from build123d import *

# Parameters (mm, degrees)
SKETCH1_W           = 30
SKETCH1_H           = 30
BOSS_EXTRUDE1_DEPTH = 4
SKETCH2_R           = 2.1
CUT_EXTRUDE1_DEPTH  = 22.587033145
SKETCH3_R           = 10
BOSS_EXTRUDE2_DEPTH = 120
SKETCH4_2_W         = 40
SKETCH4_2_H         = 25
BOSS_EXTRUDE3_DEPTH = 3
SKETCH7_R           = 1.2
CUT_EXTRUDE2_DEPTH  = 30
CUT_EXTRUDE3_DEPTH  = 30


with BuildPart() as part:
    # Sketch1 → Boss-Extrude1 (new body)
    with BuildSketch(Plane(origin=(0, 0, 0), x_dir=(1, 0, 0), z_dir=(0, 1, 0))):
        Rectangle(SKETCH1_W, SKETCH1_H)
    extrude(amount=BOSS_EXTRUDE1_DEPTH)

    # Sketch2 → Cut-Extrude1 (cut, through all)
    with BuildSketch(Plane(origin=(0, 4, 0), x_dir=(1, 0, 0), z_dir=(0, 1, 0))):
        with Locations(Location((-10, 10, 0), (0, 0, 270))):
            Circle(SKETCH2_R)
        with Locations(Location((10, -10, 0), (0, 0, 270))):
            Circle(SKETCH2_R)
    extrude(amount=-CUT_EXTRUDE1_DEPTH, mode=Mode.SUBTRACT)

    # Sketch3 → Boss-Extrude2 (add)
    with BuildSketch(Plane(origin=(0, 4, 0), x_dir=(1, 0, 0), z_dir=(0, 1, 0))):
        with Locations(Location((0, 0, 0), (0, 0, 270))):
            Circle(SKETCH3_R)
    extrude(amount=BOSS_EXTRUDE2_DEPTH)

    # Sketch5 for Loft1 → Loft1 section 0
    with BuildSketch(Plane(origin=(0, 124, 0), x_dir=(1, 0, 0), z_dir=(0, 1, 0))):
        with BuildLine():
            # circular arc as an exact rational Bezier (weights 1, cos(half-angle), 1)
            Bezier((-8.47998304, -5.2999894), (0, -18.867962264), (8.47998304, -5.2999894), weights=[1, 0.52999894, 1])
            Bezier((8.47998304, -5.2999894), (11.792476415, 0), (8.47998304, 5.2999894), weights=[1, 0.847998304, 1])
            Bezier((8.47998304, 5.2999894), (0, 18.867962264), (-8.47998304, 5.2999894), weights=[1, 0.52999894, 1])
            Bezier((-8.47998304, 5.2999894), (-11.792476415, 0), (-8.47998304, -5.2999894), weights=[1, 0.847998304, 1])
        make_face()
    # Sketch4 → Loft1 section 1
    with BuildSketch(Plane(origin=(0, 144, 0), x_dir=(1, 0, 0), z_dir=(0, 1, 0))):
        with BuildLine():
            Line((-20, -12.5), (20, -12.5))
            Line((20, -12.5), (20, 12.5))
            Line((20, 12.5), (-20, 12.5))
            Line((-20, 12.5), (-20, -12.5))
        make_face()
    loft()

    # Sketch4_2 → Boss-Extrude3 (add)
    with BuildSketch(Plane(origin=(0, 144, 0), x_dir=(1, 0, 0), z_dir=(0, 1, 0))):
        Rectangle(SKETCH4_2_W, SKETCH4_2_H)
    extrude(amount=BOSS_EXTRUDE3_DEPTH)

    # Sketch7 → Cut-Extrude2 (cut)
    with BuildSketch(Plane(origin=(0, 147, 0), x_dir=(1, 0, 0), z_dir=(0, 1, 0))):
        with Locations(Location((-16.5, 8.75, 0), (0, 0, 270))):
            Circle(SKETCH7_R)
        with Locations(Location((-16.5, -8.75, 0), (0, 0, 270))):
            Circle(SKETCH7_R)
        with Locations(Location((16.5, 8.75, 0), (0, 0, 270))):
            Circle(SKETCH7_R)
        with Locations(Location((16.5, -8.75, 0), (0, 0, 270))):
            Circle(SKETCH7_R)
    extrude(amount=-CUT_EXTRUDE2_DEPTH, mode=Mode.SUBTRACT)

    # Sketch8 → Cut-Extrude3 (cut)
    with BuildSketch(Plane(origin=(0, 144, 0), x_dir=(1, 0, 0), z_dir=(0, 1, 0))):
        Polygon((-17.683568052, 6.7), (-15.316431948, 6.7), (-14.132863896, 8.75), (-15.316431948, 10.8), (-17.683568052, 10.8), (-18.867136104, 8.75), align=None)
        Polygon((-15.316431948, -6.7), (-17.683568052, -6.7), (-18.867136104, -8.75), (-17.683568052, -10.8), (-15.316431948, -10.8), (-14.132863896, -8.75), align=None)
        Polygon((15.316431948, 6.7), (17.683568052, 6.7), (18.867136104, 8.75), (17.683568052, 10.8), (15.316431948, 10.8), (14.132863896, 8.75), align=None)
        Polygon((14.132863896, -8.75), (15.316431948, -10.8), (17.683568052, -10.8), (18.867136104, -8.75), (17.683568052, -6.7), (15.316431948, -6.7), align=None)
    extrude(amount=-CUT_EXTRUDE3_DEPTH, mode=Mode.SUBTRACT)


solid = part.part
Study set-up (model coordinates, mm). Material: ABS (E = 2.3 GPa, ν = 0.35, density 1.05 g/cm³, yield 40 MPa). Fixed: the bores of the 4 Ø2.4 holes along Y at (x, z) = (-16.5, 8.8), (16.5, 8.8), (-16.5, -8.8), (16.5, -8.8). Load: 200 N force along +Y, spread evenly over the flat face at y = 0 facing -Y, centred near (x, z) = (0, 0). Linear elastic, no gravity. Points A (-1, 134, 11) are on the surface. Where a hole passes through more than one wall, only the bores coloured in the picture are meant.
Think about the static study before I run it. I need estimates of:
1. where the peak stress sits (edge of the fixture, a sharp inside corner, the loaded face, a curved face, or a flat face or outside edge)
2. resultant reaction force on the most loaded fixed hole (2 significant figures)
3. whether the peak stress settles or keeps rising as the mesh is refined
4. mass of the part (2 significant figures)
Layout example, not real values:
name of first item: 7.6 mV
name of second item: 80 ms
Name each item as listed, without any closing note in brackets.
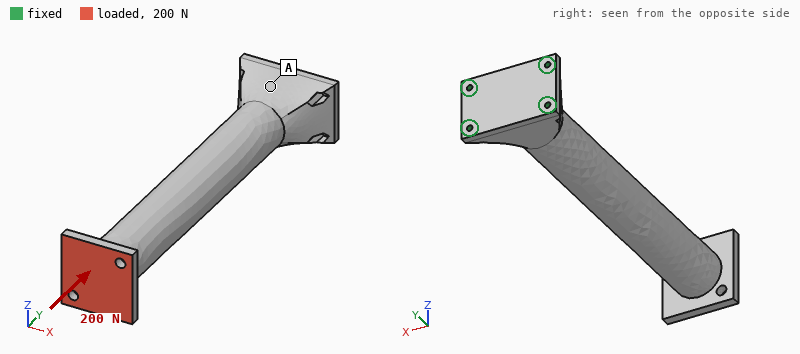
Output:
where the peak stress sits: edge of the fixture
resultant reaction force on the most loaded fixed hole: 56 N
whether the peak stress settles or keeps rising as the mesh is refined: keeps rising
mass of the part: 59 g
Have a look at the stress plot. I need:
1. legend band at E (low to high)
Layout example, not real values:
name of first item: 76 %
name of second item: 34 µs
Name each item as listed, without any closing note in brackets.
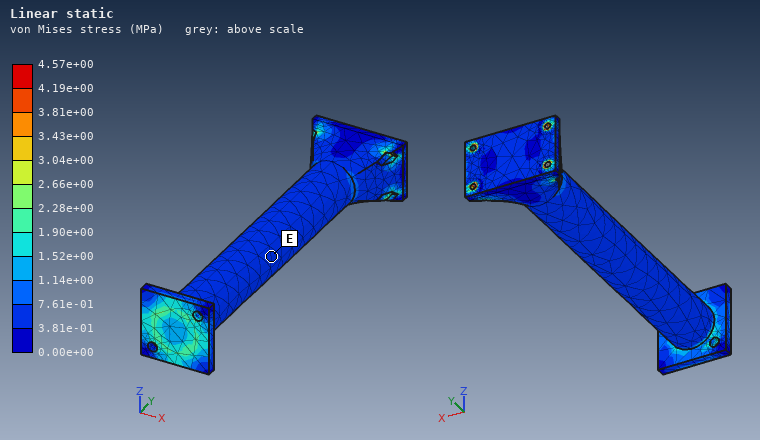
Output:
legend band at E: 3.81e-01 to 7.61e-01 MPa
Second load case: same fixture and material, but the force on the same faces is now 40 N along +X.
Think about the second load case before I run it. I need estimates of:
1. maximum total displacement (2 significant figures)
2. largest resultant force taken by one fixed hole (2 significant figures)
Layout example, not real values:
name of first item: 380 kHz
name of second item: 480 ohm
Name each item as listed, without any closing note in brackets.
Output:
maximum total displacement: 1.8 mm
largest resultant force taken by one fixed hole: 93 N
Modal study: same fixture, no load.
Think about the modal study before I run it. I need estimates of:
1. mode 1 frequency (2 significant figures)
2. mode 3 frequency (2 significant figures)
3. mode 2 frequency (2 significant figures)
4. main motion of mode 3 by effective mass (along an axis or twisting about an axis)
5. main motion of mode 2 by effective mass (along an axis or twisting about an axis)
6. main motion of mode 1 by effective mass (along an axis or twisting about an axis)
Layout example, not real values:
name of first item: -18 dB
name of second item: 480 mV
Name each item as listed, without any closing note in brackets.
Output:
mode 1 frequency: 180 Hz
mode 3 frequency: 1000 Hz
mode 2 frequency: 210 Hz
main motion of mode 3 by effective mass: along Z
main motion of mode 2 by effective mass: along X
main motion of mode 1 by effective mass: along Z
